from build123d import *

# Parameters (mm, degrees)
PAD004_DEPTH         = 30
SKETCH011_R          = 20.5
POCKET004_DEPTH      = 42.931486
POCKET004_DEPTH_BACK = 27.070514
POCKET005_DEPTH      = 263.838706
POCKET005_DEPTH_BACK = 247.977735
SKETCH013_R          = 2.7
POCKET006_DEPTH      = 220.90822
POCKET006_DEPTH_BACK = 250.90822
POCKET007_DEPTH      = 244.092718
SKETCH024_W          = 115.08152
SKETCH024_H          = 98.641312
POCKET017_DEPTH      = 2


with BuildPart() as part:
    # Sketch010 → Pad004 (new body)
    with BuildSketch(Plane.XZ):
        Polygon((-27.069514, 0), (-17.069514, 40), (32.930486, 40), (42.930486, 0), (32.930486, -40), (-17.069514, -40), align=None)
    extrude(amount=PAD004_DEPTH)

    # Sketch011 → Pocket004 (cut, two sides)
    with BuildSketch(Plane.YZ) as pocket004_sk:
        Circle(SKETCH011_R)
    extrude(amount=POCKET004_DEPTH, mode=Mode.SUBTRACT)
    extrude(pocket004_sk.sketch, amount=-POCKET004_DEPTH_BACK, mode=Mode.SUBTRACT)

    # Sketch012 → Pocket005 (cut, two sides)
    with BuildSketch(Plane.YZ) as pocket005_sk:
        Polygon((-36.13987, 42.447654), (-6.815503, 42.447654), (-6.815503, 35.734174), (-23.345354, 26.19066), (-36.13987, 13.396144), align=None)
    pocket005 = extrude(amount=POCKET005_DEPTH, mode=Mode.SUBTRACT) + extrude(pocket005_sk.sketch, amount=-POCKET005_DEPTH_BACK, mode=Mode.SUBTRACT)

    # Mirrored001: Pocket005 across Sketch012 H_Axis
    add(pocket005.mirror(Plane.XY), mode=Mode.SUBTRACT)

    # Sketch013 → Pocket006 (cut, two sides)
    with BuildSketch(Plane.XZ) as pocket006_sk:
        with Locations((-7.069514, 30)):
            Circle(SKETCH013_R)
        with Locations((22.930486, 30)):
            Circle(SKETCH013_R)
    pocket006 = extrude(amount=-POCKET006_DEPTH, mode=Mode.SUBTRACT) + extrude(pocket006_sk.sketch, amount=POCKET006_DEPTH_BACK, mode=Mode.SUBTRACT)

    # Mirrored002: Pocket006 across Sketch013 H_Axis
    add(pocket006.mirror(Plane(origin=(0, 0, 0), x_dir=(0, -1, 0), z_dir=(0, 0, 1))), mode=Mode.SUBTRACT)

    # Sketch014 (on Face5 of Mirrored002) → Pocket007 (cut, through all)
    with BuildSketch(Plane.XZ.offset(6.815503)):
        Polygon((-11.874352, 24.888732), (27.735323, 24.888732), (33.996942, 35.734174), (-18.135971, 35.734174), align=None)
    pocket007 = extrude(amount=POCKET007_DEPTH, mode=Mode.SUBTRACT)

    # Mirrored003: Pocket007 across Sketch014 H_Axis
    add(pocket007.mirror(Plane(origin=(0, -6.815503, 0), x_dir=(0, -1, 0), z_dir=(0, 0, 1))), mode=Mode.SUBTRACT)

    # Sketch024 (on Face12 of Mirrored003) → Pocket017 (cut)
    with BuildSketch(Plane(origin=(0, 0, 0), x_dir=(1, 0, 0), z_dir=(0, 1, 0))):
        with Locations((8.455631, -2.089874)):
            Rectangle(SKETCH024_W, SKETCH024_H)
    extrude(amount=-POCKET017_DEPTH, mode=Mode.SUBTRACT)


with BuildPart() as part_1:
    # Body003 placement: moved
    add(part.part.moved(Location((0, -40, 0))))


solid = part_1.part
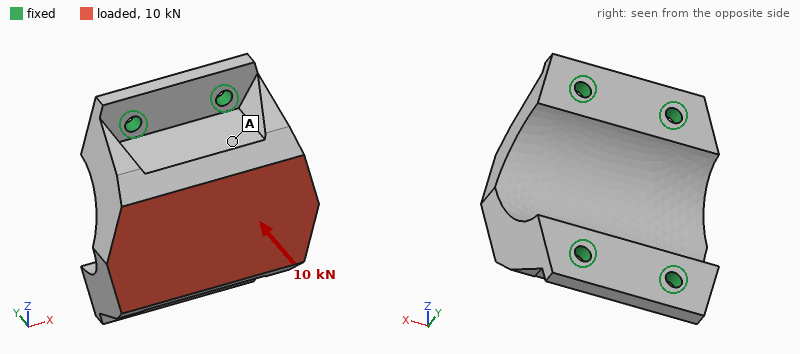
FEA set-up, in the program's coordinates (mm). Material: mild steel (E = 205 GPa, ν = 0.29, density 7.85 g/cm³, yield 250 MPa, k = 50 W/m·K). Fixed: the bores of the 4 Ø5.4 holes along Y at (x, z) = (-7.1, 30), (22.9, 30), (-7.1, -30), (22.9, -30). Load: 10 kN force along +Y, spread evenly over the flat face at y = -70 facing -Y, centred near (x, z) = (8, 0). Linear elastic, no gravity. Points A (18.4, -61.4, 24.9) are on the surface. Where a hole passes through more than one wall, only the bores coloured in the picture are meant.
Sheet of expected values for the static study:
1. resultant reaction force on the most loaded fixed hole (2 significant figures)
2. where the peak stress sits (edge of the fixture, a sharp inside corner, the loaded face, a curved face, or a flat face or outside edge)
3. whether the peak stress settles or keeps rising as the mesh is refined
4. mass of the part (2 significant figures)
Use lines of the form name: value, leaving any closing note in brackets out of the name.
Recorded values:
resultant reaction force on the most loaded fixed hole: 3.1 kN
where the peak stress sits: edge of the fixture
whether the peak stress settles or keeps rising as the mesh is refined: keeps rising
mass of the part: 460 g
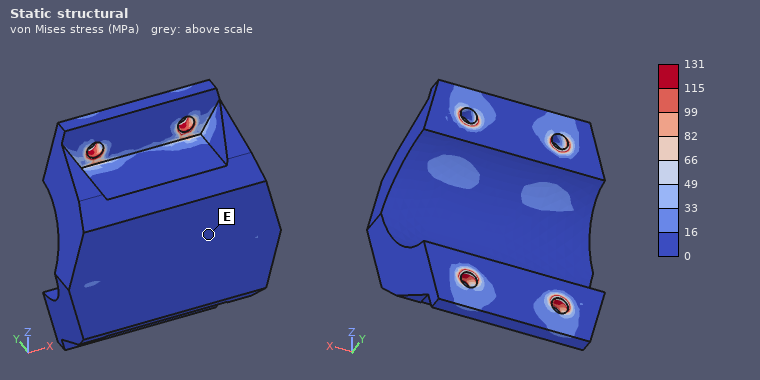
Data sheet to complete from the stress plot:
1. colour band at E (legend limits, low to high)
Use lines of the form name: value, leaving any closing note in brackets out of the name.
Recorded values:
colour band at E: 0 to 16 MPa
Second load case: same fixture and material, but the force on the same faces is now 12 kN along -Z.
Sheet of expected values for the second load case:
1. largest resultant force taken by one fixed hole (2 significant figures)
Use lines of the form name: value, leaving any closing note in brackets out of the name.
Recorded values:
largest resultant force taken by one fixed hole: 4.0 kN
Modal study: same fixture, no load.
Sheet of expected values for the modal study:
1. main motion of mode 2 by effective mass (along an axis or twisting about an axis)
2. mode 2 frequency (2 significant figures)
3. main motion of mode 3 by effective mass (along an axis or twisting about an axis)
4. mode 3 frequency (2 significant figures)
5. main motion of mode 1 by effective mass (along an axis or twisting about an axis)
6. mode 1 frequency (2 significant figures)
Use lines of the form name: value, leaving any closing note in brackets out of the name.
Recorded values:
main motion of mode 2 by effective mass: along Z
mode 2 frequency: 10 kHz
main motion of mode 3 by effective mass: along Y
mode 3 frequency: 11 kHz
main motion of mode 1 by effective mass: along X
mode 1 frequency: 6800 Hz
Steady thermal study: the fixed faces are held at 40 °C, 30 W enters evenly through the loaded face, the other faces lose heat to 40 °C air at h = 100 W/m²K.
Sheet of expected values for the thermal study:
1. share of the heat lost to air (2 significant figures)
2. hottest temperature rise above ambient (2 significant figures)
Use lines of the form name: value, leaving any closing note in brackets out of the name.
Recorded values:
share of the heat lost to air: 36 %
hottest temperature rise above ambient: 16 K
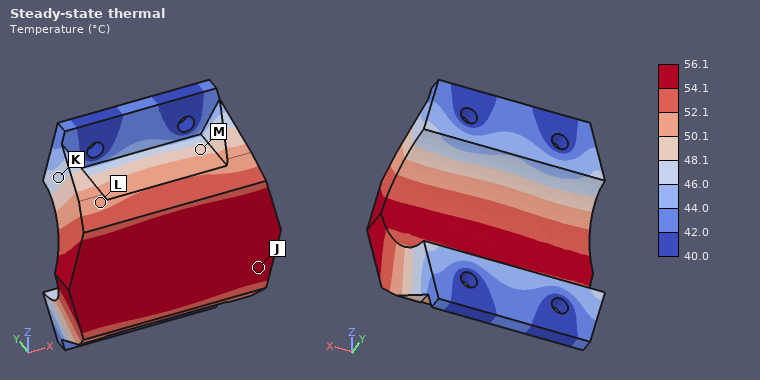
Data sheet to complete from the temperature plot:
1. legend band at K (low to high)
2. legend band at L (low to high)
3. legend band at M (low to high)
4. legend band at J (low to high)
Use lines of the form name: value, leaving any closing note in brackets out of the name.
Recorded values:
legend band at K: 46.0 to 48.1 °C
legend band at L: 50.1 to 52.1 °C
legend band at M: 48.1 to 50.1 °C
legend band at J: 54.1 to 56.1 °C
